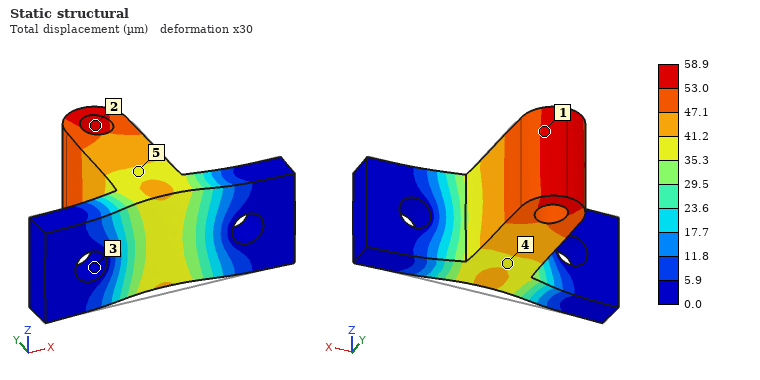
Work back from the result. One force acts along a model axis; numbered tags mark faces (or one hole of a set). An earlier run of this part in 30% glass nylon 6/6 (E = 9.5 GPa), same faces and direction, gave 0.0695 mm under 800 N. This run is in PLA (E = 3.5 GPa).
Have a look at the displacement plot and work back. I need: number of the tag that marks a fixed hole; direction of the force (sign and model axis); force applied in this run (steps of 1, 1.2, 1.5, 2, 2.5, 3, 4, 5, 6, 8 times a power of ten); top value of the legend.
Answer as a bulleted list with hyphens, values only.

- 3
- +Y
- 250 N
- 58.9 µm
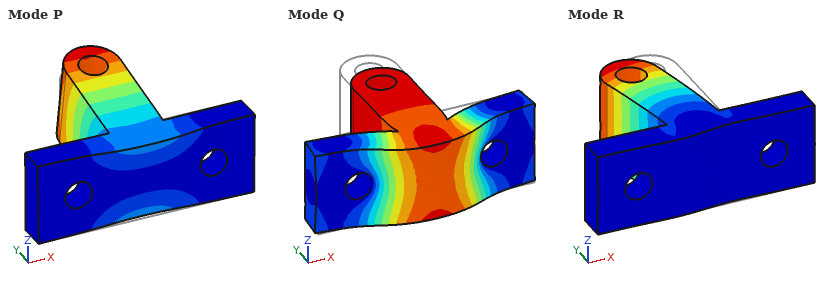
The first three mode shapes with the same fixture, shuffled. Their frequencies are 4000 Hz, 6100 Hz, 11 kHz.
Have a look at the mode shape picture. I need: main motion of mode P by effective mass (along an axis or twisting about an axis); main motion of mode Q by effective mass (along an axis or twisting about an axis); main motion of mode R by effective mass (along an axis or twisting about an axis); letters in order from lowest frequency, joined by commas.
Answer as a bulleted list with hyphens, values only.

- along Z
- along Y
- along X
- P, R, Q
